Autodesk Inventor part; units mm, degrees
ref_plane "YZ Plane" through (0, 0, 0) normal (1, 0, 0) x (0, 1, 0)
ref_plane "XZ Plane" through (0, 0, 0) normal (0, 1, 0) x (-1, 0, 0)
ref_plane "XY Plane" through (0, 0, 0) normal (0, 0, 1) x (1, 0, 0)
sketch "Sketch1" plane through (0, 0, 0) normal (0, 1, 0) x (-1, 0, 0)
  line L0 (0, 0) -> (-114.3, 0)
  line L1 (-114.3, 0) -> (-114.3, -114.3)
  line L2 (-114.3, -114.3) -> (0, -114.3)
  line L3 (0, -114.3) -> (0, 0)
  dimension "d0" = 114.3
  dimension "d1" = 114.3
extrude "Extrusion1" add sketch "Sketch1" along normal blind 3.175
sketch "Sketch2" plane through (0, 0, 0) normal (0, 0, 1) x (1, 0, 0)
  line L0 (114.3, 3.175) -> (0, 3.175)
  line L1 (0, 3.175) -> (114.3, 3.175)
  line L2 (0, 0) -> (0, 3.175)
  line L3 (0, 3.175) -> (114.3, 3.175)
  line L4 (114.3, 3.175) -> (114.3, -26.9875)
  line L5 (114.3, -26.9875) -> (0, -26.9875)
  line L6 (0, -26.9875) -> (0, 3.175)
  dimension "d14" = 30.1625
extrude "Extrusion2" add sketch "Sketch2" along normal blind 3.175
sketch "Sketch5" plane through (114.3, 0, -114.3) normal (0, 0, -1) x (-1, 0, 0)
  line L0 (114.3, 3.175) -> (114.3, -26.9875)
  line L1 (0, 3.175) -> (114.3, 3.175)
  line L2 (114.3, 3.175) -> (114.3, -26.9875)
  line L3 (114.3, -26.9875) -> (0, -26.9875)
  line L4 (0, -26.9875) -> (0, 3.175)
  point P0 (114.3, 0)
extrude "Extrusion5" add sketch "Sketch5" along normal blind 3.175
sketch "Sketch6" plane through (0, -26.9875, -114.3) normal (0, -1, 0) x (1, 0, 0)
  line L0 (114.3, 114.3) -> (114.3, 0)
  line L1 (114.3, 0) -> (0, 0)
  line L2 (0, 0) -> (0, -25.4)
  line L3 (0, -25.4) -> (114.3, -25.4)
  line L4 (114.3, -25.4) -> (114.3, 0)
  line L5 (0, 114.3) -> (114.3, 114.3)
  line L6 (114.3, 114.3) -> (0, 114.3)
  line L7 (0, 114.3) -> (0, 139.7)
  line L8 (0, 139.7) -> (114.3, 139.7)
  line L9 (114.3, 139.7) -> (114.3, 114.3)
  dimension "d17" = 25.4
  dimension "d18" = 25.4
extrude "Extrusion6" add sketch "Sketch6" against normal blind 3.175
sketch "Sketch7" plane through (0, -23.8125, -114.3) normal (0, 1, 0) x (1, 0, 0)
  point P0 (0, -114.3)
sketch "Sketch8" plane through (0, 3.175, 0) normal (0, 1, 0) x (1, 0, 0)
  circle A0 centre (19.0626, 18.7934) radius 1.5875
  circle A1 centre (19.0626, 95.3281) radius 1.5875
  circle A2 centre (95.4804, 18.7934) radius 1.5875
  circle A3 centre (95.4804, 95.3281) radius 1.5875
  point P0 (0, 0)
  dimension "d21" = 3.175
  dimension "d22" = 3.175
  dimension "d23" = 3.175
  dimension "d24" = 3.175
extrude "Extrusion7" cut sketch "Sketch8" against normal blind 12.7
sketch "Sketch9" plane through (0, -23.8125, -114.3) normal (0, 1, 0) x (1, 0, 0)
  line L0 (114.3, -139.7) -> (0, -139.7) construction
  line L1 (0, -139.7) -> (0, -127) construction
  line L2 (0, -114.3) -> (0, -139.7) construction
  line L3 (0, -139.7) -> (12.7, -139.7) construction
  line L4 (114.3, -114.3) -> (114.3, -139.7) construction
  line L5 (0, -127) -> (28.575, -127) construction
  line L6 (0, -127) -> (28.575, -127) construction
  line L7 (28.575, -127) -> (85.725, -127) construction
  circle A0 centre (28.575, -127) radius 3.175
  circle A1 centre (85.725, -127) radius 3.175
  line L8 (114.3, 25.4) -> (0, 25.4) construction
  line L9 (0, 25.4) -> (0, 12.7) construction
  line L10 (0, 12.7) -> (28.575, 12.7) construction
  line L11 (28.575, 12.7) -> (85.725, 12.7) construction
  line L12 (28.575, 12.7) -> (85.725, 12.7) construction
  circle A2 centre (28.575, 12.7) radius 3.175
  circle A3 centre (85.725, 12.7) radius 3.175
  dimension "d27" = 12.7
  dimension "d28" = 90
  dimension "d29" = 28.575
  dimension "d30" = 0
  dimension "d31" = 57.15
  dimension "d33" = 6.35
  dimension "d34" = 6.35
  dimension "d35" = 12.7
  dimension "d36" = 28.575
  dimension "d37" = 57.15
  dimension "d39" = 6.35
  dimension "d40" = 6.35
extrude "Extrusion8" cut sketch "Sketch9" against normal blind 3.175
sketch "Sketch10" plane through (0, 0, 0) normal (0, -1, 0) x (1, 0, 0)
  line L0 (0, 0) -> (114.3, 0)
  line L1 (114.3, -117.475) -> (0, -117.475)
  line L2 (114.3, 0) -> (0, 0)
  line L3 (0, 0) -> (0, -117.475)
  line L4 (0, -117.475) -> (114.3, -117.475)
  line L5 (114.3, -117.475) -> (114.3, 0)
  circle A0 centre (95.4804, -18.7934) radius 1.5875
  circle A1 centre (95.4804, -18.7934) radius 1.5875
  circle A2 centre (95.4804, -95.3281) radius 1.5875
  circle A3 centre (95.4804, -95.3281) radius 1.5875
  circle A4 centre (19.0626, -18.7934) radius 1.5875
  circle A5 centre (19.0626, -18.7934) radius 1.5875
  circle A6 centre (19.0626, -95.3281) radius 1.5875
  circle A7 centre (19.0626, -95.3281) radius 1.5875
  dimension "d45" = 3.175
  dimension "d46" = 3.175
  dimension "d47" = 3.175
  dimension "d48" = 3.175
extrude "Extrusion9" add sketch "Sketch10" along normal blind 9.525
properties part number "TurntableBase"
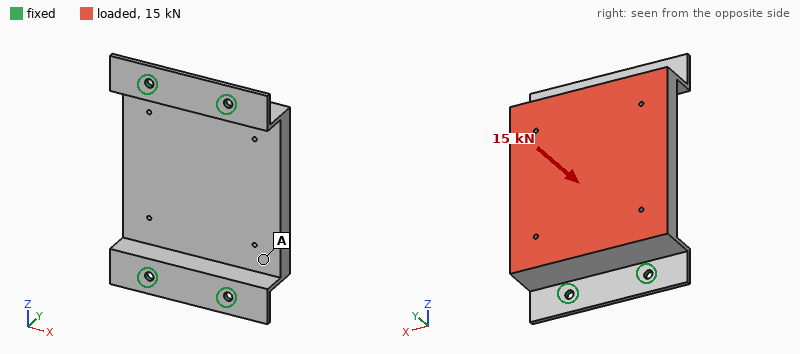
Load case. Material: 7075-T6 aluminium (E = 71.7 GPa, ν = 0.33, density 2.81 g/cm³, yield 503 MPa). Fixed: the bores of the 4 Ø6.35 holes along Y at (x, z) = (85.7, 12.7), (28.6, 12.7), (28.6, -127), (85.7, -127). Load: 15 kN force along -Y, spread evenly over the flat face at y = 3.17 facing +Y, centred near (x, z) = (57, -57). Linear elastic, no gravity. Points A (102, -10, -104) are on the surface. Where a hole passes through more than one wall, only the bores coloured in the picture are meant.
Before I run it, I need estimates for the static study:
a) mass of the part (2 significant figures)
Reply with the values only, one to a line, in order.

570 g
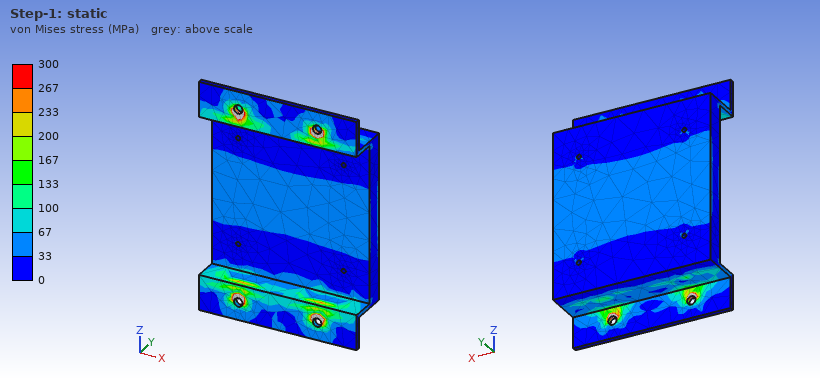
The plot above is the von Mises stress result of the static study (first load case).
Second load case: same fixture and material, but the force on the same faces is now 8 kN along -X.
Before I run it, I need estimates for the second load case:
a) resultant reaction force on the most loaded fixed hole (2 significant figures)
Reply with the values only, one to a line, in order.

3.1 kN
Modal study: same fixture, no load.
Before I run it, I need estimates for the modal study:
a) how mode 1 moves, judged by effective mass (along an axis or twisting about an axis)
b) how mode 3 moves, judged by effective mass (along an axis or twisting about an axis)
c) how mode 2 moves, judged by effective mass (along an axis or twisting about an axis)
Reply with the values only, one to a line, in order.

along Z
along Y
along X
